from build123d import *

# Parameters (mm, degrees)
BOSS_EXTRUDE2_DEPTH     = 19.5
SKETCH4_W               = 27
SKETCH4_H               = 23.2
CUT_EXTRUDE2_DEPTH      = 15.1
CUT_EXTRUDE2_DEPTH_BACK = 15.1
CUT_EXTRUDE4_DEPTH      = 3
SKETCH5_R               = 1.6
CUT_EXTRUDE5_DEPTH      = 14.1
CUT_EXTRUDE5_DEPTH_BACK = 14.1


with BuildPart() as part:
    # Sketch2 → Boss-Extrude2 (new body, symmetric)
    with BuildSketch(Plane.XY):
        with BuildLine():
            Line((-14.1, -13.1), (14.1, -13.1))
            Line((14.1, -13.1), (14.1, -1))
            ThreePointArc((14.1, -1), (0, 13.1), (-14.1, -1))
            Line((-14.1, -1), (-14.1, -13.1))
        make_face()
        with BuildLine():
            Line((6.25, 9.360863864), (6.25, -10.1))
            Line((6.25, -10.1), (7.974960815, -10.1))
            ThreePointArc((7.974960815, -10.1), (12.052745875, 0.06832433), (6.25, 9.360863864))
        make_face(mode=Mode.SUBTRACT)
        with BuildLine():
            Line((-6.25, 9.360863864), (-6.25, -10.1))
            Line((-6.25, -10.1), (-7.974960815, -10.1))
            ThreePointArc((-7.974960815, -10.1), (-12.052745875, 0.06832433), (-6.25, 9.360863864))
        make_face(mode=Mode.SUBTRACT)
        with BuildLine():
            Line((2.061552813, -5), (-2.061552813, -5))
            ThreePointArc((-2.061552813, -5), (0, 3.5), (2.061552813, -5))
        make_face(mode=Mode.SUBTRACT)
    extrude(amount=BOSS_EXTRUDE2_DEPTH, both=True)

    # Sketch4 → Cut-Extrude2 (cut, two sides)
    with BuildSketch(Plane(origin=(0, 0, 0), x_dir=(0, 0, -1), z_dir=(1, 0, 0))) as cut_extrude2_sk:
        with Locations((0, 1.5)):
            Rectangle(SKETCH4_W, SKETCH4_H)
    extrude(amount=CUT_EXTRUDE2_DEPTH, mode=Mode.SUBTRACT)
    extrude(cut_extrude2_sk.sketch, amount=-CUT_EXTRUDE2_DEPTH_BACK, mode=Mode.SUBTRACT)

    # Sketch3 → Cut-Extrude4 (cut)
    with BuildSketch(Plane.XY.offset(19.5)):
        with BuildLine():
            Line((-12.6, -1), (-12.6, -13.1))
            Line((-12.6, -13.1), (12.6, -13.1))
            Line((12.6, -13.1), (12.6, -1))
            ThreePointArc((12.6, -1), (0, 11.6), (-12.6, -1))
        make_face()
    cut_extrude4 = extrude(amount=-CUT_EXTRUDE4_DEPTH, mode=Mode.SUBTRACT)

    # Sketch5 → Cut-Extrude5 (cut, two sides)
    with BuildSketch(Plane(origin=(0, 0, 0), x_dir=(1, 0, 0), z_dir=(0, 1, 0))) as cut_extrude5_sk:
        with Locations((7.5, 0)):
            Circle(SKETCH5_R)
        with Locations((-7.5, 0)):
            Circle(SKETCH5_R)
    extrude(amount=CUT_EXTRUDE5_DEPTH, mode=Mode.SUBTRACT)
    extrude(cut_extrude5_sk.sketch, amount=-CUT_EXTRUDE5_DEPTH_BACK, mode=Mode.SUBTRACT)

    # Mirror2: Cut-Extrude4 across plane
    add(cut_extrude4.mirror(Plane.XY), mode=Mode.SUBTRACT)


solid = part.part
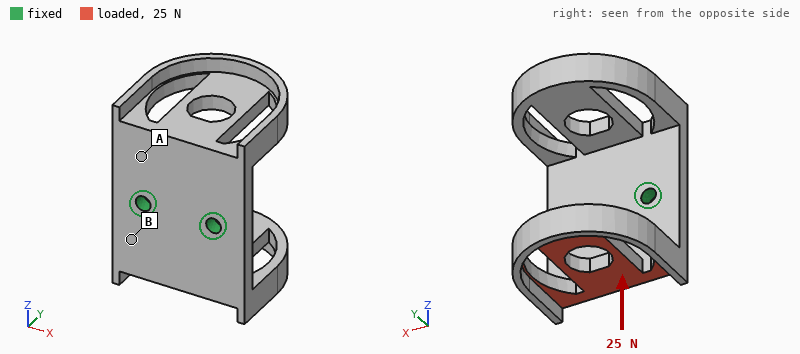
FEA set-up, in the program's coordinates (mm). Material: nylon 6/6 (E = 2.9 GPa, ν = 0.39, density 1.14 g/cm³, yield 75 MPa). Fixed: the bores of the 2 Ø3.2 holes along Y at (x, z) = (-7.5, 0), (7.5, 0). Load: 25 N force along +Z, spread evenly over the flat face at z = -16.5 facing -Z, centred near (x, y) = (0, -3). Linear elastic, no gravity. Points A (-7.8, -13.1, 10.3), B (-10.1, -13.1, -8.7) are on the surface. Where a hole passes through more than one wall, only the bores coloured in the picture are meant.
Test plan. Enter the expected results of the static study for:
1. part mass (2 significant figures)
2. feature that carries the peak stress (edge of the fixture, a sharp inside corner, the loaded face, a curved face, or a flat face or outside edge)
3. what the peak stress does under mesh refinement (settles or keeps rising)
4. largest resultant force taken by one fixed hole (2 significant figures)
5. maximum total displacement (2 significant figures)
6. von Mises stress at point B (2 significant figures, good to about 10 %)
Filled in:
6.1 g
edge of the fixture
keeps rising
13 N
0.62 mm
4.7 MPa
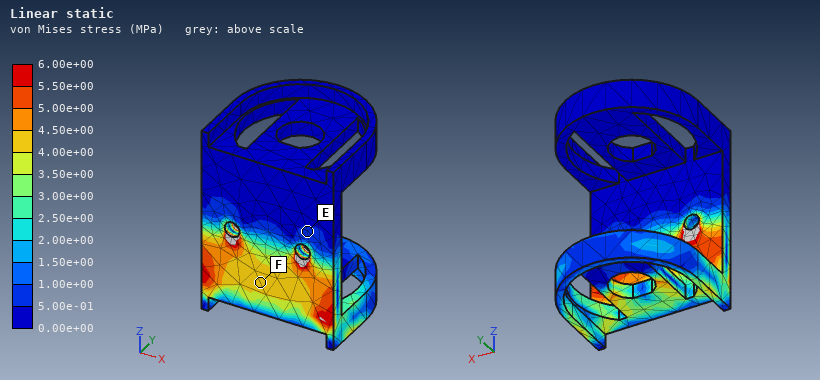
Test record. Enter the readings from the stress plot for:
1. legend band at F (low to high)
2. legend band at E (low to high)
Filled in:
4.00e+00 to 4.50e+00 MPa
5.00e-01 to 1.00e+00 MPa
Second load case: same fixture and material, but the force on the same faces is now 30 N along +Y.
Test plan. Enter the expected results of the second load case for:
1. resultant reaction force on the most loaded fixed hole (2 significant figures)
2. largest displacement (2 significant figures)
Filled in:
15 N
0.60 mm
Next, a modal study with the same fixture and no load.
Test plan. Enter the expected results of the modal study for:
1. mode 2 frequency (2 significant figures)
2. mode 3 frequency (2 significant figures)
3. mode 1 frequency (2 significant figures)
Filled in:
780 Hz
1300 Hz
760 Hz
